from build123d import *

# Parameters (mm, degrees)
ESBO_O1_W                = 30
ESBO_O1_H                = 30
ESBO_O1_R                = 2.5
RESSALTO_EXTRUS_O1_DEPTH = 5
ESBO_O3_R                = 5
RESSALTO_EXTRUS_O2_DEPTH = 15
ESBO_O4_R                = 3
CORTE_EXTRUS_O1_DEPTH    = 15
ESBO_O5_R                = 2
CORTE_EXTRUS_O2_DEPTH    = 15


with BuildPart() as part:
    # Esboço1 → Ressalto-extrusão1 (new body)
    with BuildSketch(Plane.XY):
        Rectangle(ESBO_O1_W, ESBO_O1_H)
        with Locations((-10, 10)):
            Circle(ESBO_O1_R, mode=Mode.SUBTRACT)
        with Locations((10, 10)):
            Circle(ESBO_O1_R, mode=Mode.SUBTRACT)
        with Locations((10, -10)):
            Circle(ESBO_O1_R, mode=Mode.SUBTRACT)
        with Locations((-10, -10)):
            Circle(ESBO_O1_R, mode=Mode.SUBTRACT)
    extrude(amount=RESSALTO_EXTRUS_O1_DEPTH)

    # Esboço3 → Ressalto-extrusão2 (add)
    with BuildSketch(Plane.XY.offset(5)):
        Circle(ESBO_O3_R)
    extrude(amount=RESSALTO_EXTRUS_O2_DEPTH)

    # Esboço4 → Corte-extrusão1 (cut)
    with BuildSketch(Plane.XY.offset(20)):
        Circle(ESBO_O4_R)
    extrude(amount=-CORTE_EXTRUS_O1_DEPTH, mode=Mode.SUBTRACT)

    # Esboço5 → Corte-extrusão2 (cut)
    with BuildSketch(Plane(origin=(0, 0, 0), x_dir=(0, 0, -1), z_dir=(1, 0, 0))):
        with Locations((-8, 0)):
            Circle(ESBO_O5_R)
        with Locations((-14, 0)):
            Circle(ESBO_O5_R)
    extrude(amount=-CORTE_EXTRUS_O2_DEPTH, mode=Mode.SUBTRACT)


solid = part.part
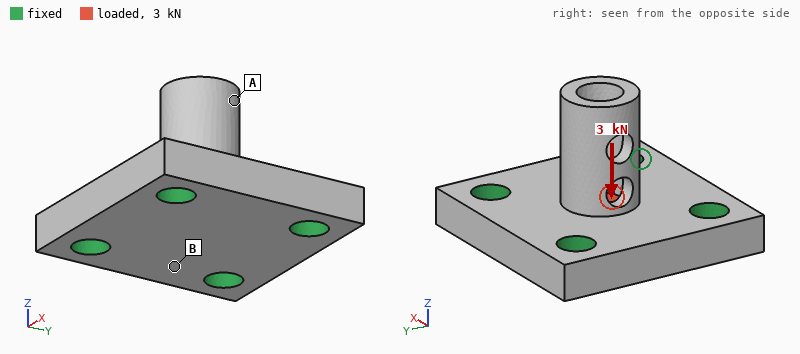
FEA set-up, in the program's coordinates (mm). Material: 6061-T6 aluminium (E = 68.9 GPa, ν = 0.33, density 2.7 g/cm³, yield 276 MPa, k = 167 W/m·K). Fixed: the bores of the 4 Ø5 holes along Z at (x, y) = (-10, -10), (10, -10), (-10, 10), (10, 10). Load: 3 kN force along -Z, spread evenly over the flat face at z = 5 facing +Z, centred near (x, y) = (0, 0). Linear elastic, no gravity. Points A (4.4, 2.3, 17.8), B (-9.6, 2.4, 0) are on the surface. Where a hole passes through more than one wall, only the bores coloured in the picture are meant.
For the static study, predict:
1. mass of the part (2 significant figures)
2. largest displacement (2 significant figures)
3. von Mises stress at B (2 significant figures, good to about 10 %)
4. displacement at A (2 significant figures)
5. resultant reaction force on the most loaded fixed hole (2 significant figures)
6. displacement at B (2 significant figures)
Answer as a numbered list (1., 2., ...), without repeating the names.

1. 13 g
2. 21 µm
3. 26 MPa
4. 13 µm
5. 760 N
6. 5.2 µm
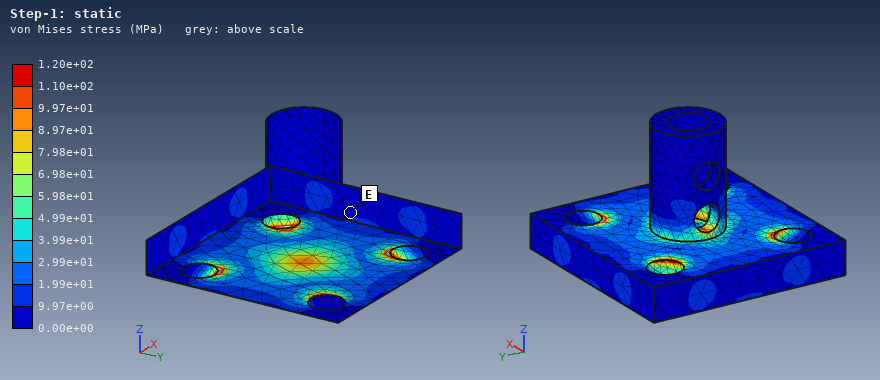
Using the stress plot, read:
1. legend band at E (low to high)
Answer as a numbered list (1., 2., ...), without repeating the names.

1. 0.00e+00 to 9.97e+00 MPa
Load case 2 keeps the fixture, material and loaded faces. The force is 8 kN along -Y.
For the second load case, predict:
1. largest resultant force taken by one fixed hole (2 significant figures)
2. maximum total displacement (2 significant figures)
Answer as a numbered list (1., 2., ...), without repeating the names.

1. 2.3 kN
2. 30 µm
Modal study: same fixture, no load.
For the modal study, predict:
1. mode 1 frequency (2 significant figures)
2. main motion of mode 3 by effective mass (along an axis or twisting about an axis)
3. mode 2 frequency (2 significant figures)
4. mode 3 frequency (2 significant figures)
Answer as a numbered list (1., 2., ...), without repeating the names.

1. 19 kHz
2. along Z
3. 19 kHz
4. 36 kHz
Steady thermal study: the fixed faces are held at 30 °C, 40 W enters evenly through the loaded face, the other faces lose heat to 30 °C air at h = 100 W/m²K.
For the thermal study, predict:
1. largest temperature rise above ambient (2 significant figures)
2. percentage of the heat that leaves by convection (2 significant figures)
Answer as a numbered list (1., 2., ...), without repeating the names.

1. 26 K
2. 3.5 %
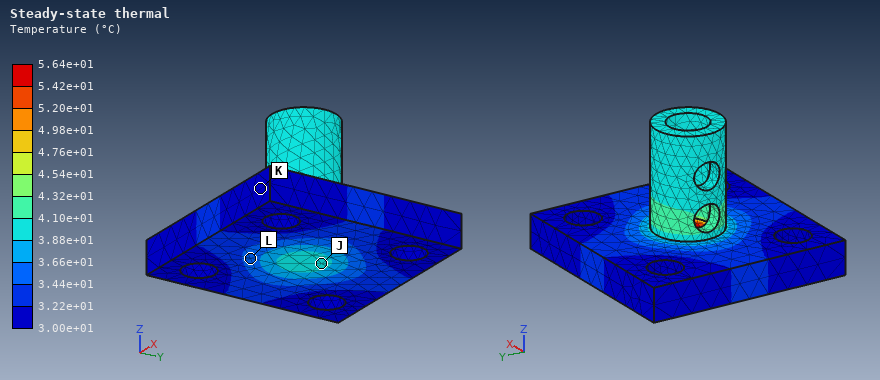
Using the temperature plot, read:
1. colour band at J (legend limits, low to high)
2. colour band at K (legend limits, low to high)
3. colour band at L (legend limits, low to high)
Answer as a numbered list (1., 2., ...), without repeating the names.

1. 3.88e+01 to 4.10e+01 °C
2. 3.00e+01 to 3.22e+01 °C
3. 3.44e+01 to 3.66e+01 °C
